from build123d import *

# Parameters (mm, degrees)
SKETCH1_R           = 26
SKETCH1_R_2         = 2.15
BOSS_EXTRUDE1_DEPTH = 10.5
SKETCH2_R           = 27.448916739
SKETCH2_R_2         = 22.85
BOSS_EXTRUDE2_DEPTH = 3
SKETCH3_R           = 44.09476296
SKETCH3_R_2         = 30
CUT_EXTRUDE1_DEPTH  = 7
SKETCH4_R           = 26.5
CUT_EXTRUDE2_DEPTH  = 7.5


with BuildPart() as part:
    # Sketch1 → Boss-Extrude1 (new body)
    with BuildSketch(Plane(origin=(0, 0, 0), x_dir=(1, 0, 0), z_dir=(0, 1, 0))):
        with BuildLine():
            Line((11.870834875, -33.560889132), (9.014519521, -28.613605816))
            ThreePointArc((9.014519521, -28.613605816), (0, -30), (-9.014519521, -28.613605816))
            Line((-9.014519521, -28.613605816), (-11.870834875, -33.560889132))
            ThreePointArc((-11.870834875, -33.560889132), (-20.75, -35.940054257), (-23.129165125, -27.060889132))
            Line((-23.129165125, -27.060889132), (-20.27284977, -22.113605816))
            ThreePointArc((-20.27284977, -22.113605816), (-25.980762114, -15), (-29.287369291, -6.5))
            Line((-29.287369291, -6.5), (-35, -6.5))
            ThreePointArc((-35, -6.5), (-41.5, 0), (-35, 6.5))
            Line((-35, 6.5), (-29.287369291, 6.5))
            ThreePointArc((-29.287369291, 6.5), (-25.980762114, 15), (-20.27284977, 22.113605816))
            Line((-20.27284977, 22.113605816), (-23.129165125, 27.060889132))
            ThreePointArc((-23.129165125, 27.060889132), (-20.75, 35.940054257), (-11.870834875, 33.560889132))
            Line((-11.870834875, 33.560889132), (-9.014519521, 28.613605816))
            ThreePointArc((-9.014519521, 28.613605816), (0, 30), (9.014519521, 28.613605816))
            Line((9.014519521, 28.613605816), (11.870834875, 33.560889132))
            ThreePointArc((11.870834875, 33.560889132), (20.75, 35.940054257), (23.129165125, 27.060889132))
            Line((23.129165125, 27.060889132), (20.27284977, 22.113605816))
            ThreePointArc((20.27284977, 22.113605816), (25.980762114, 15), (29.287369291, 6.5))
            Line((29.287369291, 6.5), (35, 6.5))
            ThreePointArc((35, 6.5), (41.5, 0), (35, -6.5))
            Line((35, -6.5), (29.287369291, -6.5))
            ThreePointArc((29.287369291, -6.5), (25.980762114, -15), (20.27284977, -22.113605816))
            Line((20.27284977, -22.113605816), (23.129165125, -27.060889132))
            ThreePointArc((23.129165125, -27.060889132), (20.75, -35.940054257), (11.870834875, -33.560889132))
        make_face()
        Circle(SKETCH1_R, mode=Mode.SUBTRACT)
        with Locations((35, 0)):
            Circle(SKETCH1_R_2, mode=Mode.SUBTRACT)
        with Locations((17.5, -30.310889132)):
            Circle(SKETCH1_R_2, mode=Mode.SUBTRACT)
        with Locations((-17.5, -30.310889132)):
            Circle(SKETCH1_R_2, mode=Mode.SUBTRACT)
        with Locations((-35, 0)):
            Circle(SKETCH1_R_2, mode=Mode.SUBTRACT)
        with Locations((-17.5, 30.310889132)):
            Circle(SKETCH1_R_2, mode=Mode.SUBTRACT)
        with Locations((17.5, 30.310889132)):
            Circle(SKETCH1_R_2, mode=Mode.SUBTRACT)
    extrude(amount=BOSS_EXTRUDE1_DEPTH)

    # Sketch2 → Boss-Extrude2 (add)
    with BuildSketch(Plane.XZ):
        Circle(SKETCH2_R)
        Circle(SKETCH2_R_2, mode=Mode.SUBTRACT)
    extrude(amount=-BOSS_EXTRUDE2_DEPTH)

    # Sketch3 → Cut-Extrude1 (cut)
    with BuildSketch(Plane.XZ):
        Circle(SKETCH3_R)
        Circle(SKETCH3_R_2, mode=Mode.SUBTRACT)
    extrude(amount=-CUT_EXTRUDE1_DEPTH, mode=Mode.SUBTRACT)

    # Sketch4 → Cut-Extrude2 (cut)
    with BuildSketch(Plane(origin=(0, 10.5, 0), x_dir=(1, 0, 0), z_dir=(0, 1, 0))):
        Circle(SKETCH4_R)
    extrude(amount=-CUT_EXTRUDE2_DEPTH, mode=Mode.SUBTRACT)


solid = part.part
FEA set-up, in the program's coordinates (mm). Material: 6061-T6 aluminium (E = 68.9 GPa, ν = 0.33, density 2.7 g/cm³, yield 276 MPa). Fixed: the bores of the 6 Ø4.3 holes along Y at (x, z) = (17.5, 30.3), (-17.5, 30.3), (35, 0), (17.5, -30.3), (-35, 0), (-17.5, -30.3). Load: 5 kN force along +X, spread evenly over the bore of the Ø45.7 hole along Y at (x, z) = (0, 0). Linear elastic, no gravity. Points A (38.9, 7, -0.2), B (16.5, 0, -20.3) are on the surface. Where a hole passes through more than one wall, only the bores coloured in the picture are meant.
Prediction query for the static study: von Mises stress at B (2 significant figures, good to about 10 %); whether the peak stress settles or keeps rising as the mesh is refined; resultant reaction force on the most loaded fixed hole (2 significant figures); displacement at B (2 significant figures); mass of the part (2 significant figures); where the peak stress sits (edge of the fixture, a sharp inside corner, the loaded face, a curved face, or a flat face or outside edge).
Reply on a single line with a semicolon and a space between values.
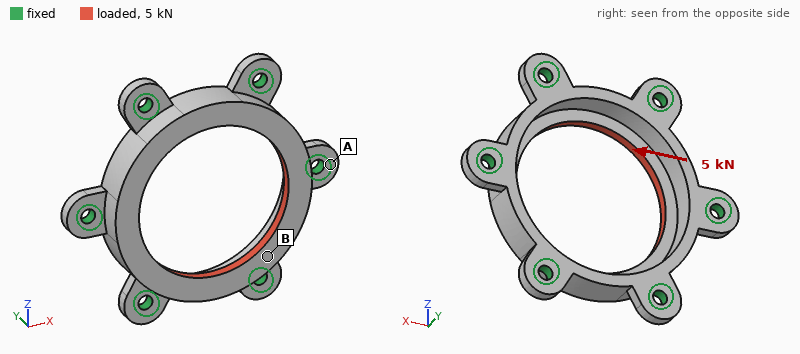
25 MPa; keeps rising; 940 N; 20 µm; 29 g; edge of the fixture
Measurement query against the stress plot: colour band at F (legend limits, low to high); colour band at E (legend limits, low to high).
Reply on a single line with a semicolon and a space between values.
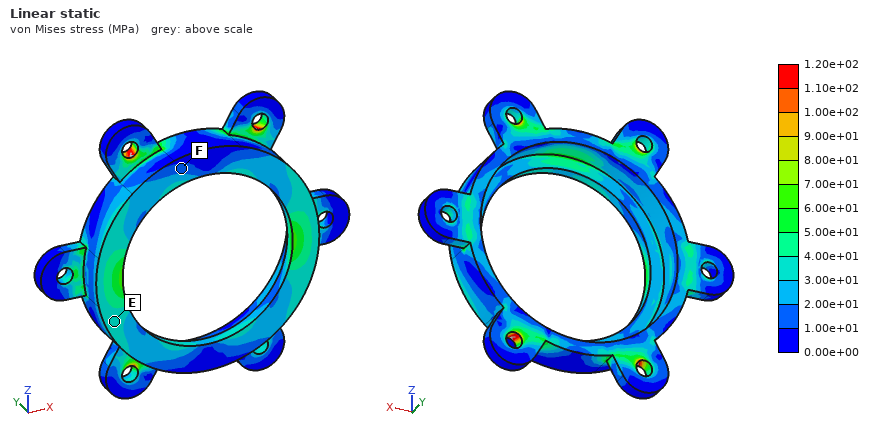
1.00e+01 to 2.00e+01 MPa; 3.00e+01 to 4.00e+01 MPa
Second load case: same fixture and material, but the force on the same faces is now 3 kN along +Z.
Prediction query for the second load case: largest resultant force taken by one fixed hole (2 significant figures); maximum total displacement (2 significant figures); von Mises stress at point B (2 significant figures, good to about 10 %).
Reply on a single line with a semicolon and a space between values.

600 N; 20 µm; 24 MPa
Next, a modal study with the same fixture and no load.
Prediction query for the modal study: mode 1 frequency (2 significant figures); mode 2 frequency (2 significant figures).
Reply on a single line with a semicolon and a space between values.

18 kHz; 18 kHz
